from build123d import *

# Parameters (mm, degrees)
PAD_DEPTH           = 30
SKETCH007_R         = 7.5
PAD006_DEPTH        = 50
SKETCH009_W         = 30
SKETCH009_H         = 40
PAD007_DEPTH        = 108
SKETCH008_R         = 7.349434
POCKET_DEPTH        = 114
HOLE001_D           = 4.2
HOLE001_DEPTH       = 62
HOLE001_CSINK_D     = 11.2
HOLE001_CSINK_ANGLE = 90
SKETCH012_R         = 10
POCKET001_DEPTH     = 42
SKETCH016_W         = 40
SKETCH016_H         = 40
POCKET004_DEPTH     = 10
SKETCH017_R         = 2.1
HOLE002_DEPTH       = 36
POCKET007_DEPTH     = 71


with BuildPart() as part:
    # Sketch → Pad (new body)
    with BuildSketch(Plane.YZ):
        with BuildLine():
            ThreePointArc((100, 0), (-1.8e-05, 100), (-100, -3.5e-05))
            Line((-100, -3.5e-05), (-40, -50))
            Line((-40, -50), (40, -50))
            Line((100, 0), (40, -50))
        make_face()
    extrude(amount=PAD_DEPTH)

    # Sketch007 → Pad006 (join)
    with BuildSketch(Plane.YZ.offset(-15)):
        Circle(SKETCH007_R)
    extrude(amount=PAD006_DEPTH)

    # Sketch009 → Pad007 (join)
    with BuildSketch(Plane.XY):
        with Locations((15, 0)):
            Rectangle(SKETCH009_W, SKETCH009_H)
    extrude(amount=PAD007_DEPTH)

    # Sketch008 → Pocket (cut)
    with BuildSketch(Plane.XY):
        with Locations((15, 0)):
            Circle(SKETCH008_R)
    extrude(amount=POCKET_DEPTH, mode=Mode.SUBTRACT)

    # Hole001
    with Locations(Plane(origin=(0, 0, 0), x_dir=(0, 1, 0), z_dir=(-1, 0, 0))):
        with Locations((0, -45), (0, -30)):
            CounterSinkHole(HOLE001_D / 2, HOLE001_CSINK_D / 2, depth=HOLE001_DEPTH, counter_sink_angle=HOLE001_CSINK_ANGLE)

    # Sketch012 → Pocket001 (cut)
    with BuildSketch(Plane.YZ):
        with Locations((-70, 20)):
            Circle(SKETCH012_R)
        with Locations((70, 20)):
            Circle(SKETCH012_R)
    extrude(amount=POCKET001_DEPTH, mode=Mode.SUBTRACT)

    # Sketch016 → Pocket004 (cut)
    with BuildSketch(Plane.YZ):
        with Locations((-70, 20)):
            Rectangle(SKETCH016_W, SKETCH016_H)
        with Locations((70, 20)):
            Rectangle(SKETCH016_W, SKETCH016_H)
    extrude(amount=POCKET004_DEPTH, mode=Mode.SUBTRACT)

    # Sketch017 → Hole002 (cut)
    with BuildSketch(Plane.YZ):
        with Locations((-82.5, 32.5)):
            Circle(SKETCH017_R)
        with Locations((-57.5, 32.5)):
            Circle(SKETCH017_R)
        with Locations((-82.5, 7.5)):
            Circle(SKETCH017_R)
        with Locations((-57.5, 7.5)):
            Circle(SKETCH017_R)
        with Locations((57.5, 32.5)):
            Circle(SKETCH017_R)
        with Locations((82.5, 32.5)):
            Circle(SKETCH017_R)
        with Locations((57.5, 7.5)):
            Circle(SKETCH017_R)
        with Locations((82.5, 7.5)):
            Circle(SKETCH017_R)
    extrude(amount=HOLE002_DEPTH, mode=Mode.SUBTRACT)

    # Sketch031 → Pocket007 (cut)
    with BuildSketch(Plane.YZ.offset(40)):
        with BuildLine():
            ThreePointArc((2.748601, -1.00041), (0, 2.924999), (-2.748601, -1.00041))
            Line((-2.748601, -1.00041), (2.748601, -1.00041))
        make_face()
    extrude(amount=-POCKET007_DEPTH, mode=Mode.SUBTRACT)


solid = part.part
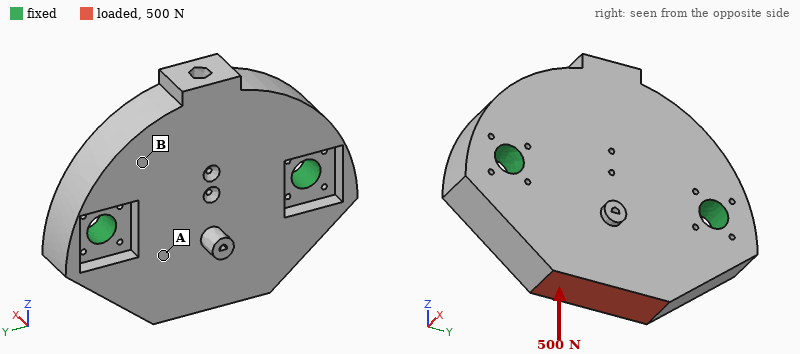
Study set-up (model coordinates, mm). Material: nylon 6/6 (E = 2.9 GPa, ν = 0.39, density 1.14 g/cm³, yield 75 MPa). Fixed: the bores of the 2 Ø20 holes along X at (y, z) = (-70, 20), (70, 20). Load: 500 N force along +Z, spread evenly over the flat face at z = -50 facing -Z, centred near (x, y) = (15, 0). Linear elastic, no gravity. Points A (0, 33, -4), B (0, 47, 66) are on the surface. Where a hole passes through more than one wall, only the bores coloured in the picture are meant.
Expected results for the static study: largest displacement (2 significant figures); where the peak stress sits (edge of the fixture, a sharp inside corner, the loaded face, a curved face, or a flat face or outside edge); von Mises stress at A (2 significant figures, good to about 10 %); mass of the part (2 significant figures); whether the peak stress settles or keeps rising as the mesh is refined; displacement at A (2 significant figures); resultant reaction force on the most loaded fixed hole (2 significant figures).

14 µm
a sharp inside corner
0.18 MPa
720 g
keeps rising
7.1 µm
260 N
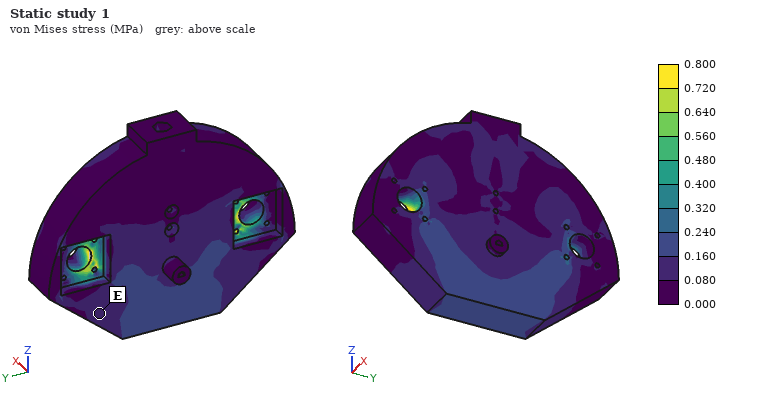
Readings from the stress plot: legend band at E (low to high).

0.080 to 0.160 MPa
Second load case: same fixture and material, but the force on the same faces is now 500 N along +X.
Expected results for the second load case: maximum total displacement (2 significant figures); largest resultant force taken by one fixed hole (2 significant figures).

0.19 mm
290 N
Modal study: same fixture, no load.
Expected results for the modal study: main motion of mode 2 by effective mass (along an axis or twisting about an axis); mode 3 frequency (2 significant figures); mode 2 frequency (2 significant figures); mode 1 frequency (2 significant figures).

along X
2000 Hz
1100 Hz
710 Hz
